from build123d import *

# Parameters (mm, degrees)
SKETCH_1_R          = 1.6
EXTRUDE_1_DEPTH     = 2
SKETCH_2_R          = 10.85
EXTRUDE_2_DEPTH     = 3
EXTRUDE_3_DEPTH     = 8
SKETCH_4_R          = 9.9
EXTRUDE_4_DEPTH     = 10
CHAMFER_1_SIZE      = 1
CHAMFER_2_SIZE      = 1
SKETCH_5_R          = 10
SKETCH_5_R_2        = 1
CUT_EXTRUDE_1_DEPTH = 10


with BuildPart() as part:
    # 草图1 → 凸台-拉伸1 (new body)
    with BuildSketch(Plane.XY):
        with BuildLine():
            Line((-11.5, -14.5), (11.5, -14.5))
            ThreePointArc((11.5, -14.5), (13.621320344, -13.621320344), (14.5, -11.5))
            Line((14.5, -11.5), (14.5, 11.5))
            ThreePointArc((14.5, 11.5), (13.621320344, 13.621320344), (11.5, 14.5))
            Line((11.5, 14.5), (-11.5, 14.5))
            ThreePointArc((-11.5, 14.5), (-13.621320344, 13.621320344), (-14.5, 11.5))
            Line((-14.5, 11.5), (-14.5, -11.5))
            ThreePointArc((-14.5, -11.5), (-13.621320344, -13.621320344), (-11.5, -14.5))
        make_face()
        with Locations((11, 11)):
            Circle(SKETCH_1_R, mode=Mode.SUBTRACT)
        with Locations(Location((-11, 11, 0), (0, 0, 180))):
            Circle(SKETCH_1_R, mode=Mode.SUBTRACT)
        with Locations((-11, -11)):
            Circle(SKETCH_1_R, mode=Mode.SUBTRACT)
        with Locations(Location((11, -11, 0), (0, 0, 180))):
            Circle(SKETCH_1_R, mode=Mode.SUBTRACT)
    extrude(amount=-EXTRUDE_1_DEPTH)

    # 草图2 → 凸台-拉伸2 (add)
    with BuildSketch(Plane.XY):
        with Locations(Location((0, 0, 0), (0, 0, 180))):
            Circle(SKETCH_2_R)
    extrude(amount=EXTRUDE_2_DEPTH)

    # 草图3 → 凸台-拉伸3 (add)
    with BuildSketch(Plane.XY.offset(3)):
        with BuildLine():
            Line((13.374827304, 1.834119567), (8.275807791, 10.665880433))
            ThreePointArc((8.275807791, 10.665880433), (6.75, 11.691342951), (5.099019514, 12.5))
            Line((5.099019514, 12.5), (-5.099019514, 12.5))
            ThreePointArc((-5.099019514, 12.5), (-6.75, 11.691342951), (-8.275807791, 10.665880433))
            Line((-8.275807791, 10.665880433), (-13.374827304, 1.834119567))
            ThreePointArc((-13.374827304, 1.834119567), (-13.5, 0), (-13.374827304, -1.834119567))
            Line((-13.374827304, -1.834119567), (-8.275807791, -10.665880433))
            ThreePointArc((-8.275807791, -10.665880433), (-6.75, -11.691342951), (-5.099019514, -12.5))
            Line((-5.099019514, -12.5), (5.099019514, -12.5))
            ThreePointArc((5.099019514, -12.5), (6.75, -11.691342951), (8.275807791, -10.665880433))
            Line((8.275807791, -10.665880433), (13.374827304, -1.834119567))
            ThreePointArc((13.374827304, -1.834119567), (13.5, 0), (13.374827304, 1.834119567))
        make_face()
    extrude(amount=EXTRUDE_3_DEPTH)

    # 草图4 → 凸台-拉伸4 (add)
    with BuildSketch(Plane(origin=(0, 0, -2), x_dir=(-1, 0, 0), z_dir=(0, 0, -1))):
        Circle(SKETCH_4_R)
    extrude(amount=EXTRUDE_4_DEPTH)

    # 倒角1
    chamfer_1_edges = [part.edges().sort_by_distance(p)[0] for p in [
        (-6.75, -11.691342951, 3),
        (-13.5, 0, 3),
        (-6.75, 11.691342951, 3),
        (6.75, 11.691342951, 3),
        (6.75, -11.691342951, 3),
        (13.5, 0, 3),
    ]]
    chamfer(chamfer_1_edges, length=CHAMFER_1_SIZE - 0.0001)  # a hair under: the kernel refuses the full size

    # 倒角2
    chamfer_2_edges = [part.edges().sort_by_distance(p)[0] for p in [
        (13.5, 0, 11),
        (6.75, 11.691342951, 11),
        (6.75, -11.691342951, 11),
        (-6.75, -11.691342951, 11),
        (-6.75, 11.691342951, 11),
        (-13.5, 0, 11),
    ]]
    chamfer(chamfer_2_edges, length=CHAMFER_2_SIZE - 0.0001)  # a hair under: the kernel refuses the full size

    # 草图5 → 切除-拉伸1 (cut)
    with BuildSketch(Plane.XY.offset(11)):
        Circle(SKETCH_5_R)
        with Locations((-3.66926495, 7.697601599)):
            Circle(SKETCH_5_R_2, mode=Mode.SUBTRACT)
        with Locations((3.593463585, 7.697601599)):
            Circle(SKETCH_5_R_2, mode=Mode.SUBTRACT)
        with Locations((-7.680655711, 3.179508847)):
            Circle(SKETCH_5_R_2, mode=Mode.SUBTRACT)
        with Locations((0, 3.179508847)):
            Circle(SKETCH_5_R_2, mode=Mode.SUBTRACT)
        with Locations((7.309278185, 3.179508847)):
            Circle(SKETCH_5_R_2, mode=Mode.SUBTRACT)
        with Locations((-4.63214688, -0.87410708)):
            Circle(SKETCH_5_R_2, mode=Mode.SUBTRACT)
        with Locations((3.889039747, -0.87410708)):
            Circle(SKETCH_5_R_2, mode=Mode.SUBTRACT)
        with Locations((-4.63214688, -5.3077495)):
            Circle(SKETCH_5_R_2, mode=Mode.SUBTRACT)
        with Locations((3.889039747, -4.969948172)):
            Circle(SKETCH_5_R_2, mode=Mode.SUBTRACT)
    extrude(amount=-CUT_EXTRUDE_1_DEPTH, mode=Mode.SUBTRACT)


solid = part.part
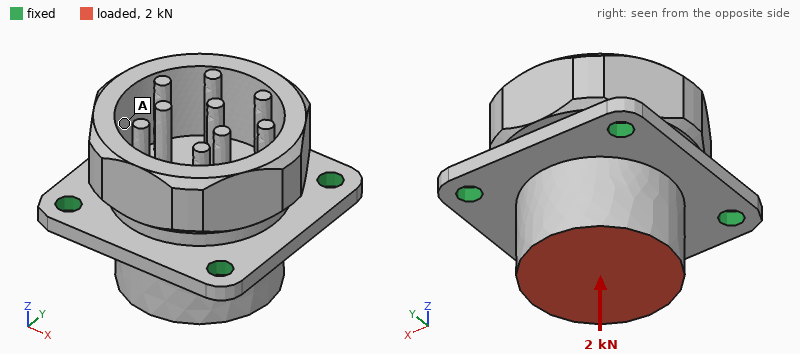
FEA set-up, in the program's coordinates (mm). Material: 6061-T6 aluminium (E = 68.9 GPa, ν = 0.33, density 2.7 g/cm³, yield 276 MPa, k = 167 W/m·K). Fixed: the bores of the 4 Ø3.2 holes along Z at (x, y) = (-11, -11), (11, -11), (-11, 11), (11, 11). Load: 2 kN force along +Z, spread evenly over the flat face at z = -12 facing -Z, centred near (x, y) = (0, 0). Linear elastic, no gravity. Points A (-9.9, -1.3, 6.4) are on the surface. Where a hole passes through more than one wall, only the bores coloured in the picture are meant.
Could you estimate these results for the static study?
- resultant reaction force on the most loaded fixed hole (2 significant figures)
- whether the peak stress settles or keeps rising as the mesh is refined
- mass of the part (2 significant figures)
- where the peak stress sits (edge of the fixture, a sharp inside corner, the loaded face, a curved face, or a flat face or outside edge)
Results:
500 N
keeps rising
19 g
edge of the fixture
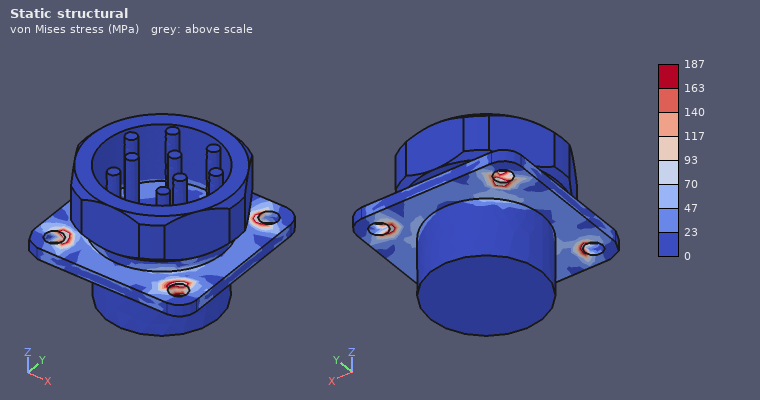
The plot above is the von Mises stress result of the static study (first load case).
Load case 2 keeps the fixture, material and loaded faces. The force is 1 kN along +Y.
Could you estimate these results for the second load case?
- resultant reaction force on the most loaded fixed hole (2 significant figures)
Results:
390 N
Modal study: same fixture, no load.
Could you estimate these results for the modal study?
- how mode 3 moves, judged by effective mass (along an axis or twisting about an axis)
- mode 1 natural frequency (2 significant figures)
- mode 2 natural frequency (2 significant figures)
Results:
along Z
12 kHz
12 kHz
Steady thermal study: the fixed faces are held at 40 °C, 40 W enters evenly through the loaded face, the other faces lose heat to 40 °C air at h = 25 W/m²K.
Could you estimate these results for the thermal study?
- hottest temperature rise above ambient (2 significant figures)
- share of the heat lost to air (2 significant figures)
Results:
24 K
3.7 %
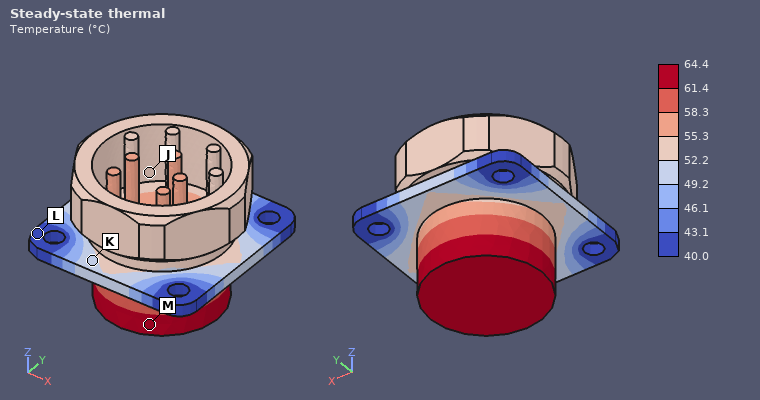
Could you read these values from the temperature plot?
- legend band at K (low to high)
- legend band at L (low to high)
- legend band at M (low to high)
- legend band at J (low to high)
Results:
49.2 to 52.2 °C
40.0 to 43.1 °C
61.4 to 64.4 °C
52.2 to 55.3 °C
